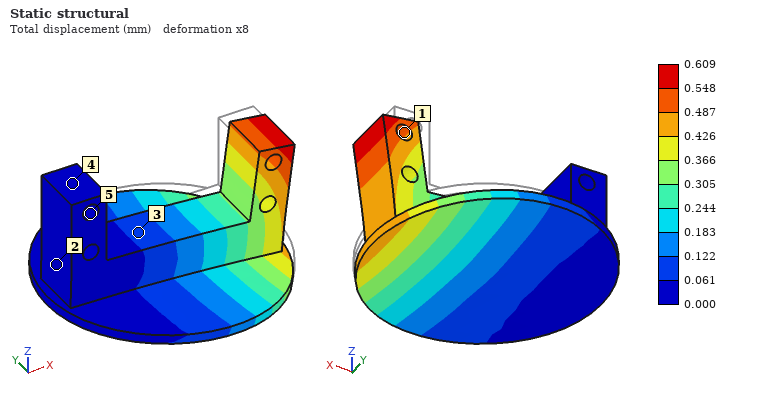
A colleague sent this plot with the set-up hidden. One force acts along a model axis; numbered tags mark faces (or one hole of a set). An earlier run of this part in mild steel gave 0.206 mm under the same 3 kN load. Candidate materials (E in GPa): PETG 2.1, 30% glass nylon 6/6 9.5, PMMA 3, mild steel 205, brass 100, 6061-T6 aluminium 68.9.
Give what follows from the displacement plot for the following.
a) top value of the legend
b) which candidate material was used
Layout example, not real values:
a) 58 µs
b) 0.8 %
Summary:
a) 0.609 mm
b) 6061-T6 aluminium
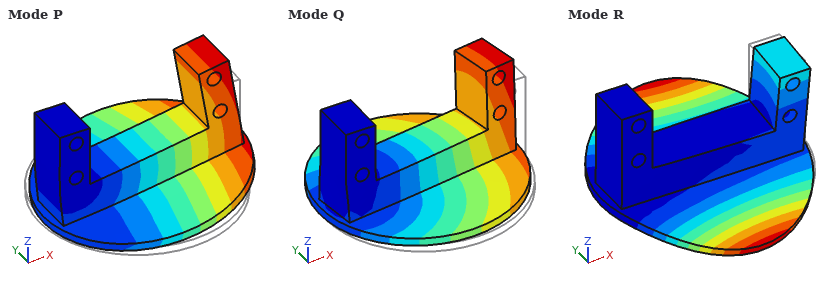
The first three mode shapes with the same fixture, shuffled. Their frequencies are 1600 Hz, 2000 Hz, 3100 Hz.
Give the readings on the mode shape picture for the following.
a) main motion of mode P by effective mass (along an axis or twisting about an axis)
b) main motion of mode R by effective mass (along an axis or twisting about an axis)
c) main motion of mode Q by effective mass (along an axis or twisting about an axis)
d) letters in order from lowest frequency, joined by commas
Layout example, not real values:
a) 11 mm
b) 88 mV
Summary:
a) along Z
b) twisting about X
c) along Y
d) P, Q, R
